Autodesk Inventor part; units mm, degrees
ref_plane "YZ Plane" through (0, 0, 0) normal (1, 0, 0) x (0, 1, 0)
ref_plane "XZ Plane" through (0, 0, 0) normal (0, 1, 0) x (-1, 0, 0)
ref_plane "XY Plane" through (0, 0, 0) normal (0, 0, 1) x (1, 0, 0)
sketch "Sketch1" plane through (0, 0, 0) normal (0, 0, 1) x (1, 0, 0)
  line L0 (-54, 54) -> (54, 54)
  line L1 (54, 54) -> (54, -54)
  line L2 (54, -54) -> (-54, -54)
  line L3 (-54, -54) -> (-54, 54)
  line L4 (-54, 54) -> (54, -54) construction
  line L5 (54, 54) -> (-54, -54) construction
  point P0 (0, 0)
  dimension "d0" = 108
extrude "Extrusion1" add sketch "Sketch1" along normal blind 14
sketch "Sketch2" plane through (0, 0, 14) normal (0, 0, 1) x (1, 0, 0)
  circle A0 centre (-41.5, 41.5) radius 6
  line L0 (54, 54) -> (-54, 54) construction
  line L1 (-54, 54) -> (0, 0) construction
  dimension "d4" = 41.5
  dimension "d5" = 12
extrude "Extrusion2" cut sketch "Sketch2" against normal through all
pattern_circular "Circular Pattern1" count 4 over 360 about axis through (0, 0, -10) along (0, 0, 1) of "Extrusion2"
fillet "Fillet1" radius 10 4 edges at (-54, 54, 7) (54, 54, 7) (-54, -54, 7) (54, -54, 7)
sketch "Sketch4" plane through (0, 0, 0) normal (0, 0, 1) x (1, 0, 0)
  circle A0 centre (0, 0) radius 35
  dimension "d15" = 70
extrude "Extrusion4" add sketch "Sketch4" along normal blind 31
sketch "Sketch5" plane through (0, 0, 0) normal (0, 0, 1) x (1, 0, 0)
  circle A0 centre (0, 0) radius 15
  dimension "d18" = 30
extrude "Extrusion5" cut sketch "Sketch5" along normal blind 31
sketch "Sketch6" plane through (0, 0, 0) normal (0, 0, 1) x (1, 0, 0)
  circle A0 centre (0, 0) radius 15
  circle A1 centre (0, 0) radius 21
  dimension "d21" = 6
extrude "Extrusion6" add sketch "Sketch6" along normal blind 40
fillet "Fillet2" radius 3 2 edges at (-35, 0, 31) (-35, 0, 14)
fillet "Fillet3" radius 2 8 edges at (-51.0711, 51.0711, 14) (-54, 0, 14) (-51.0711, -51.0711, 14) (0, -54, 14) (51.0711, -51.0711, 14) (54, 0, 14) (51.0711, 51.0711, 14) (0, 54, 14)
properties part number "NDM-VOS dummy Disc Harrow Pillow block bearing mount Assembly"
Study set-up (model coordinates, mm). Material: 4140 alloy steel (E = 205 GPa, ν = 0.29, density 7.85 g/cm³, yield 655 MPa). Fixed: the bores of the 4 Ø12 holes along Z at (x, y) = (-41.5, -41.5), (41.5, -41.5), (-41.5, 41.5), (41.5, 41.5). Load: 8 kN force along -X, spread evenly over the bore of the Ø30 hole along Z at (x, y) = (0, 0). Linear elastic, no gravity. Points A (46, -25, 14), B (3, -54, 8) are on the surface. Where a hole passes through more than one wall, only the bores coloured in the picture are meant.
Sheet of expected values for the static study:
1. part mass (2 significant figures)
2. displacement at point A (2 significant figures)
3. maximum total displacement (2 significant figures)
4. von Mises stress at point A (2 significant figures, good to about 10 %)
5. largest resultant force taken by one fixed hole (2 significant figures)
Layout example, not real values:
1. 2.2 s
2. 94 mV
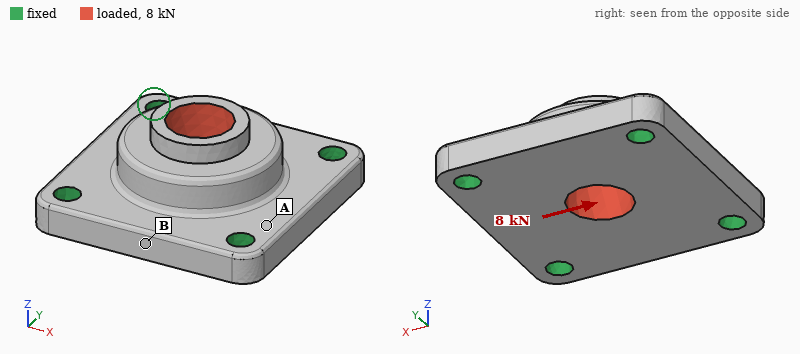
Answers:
1. 1.6 kg
2. 0.69 µm
3. 3.1 µm
4. 3.8 MPa
5. 2.3 kN
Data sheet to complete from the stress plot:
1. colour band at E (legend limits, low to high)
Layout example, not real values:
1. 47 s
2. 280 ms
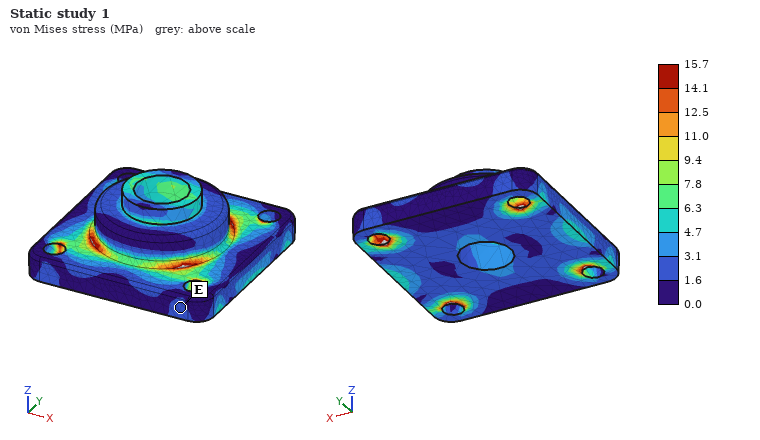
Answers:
1. 1.6 to 3.1 MPa
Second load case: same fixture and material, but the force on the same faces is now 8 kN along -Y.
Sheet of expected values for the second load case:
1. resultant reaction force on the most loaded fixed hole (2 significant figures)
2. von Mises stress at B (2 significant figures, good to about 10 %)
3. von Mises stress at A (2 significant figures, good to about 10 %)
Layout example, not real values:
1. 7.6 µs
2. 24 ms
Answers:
1. 2.3 kN
2. 3.0 MPa
3. 3.9 MPa
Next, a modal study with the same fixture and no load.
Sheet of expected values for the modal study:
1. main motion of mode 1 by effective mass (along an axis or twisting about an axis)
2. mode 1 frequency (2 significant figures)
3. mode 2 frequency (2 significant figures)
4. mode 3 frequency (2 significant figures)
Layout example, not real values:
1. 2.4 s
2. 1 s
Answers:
1. along Z
2. 7300 Hz
3. 9800 Hz
4. 9800 Hz
